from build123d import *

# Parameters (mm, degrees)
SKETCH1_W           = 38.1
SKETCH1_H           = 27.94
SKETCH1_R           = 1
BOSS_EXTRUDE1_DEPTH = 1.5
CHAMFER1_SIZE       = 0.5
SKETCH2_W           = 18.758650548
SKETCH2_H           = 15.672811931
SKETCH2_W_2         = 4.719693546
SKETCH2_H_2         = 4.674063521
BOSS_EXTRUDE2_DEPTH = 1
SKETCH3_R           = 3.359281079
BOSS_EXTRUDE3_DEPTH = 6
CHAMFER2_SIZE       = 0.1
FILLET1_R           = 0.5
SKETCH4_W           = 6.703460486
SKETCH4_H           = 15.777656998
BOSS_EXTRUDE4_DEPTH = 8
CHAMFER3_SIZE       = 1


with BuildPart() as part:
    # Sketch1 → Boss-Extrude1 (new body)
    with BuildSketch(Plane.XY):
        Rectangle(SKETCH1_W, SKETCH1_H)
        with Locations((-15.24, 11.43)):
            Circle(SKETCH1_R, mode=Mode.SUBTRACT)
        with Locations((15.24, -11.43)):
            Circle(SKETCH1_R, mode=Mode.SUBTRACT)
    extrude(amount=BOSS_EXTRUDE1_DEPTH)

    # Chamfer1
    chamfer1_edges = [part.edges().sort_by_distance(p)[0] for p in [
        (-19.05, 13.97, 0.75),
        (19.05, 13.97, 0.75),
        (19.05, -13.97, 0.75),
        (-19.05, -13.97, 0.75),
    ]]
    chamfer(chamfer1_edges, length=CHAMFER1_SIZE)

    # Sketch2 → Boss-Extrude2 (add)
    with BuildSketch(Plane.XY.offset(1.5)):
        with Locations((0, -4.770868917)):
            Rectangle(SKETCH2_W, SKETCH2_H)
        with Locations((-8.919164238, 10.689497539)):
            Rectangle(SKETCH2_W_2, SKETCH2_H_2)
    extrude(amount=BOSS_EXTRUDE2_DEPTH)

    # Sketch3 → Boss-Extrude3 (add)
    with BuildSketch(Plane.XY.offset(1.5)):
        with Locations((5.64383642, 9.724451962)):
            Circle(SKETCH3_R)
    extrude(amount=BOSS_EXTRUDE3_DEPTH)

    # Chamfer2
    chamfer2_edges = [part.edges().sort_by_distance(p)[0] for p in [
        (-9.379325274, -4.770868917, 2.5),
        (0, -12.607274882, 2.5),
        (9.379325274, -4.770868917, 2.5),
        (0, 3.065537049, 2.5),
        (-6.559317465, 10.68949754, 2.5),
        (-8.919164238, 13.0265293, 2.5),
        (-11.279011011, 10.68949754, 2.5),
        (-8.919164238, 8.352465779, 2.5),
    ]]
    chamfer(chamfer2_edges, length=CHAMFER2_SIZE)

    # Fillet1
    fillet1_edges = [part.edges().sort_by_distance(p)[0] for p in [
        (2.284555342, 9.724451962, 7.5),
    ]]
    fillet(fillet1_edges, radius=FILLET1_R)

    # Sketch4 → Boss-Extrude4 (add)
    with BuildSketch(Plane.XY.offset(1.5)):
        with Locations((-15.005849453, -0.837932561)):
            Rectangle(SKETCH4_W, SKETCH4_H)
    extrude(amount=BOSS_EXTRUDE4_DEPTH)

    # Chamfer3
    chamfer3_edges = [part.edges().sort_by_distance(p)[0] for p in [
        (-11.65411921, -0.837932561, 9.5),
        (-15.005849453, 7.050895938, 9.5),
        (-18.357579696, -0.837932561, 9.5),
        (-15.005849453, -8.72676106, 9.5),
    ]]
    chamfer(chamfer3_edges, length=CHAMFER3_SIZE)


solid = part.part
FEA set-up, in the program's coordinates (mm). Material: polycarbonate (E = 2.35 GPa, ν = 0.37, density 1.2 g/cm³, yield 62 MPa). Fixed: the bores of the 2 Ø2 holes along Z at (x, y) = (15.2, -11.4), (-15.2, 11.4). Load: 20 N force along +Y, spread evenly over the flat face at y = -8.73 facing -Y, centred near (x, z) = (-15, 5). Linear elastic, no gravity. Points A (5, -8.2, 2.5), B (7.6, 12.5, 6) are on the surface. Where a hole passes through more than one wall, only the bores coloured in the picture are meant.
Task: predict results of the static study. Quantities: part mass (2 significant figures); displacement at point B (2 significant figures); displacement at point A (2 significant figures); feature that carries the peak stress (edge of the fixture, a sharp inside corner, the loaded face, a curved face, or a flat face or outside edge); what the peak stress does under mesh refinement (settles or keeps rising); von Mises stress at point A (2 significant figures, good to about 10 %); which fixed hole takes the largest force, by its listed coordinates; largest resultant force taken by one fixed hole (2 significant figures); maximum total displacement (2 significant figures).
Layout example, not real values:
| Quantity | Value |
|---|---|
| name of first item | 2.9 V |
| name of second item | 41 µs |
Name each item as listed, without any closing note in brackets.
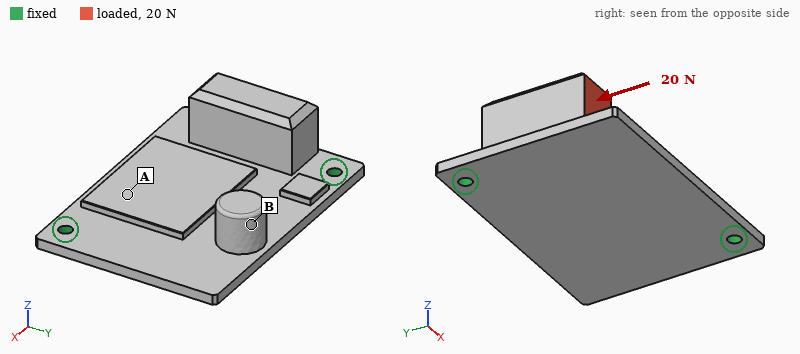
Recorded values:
| Quantity | Value |
|---|---|
| part mass | 3.5 g |
| displacement at point B | 0.23 mm |
| displacement at point A | 0.093 mm |
| feature that carries the peak stress | edge of the fixture |
| what the peak stress does under mesh refinement | keeps rising |
| von Mises stress at point A | 2.4 MPa |
| which fixed hole takes the largest force, by its listed coordinates | (-15.2, 11.4) |
| largest resultant force taken by one fixed hole | 17 N |
| maximum total displacement | 0.52 mm |
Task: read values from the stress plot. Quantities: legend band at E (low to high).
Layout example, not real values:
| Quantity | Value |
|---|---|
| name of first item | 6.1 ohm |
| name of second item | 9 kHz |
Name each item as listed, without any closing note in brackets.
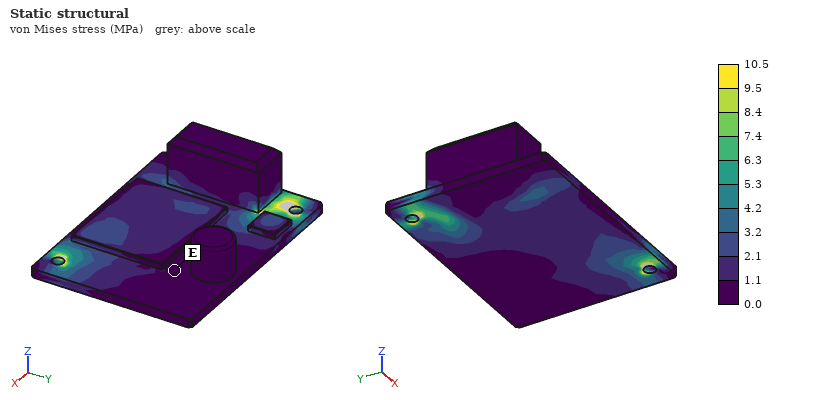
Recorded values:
| Quantity | Value |
|---|---|
| legend band at E | 0.0 to 1.1 MPa |
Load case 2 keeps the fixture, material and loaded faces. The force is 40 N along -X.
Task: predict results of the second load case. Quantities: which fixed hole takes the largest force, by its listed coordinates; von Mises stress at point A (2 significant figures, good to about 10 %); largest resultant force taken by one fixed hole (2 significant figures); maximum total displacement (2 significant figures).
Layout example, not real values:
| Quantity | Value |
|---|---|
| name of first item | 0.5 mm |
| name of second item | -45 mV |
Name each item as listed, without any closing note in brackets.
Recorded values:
| Quantity | Value |
|---|---|
| which fixed hole takes the largest force, by its listed coordinates | (15.2, -11.4) |
| von Mises stress at point A | 2.1 MPa |
| largest resultant force taken by one fixed hole | 28 N |
| maximum total displacement | 0.49 mm |
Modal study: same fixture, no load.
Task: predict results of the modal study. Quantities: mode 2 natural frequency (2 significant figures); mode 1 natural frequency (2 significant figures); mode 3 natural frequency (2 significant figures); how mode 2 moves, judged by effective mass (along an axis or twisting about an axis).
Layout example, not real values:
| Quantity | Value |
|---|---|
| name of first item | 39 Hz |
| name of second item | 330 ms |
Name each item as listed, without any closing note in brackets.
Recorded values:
| Quantity | Value |
|---|---|
| mode 2 natural frequency | 880 Hz |
| mode 1 natural frequency | 540 Hz |
| mode 3 natural frequency | 1800 Hz |
| how mode 2 moves, judged by effective mass | along Z |
